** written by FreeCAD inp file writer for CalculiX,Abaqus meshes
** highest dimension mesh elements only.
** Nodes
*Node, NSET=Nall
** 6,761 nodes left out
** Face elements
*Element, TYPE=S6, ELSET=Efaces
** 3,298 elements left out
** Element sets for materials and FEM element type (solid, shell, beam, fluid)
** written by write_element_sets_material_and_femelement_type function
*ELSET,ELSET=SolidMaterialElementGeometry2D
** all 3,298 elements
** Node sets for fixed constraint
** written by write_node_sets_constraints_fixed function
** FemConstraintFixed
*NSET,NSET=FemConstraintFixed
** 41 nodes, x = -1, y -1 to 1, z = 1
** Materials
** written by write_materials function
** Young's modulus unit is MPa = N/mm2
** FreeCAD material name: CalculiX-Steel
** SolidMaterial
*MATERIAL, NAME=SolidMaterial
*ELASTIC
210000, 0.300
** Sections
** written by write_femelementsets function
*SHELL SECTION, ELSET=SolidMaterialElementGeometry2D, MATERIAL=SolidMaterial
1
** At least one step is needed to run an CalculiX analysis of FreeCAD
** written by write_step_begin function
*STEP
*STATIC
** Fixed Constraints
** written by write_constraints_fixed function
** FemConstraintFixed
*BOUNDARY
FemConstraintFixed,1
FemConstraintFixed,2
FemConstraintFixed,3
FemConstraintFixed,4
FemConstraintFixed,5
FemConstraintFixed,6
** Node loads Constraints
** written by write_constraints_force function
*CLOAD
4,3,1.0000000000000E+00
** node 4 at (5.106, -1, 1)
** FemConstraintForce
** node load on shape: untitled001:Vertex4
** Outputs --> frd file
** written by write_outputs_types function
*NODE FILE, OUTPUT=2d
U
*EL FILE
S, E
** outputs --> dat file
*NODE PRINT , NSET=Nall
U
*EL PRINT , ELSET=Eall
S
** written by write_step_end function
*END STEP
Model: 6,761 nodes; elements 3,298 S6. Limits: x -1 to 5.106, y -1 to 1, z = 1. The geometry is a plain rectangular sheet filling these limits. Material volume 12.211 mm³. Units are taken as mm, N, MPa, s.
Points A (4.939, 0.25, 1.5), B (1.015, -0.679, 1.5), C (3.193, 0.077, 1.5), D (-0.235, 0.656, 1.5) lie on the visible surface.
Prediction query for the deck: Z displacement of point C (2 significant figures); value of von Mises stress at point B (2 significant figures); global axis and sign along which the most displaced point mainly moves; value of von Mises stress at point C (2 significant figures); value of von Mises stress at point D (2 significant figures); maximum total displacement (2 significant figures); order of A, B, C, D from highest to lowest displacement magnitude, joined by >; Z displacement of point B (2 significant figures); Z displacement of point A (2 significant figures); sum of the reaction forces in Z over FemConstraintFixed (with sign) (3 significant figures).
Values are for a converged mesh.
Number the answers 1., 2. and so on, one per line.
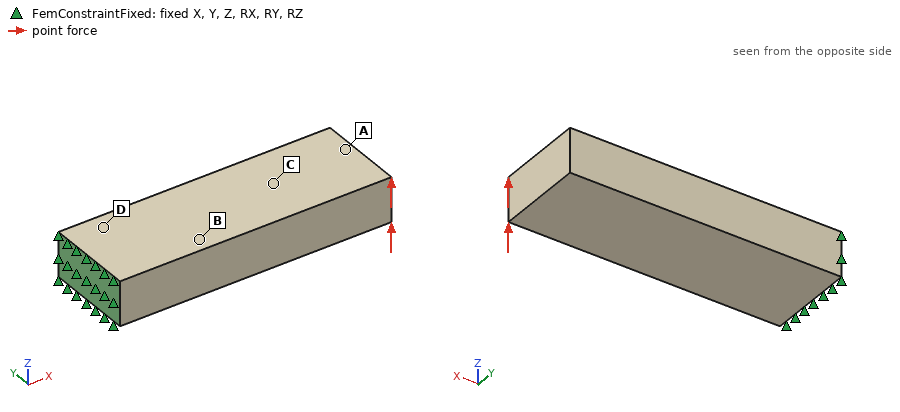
1. 0.0012 mm
2. 13 MPa
3. +Z
4. 6.6 MPa
5. 15 MPa
6. 0.0024 mm
7. A > C > B > D
8. 3.5e-04 mm
9. 0.0020 mm
10. -1.00 N
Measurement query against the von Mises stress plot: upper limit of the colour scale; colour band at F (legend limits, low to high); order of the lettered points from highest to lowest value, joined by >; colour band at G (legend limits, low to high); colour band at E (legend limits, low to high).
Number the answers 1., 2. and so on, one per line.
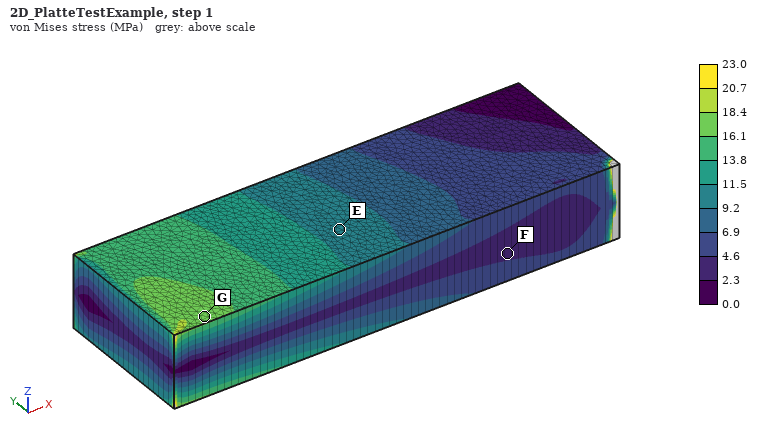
1. 23.0 MPa
2. 2.3 to 4.6 MPa
3. G > E > F
4. 16.1 to 18.4 MPa
5. 9.2 to 11.5 MPa
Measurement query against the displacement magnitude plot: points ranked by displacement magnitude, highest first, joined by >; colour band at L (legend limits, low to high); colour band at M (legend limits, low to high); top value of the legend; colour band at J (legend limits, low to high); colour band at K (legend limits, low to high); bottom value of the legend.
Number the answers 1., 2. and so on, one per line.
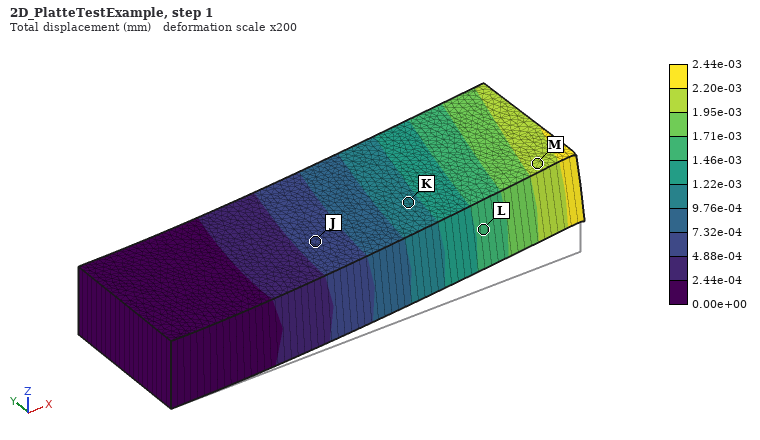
1. M > L > K > J
2. 1.46e-03 to 1.71e-03 mm
3. 1.95e-03 to 2.20e-03 mm
4. 2.44e-03 mm
5. 4.88e-04 to 7.32e-04 mm
6. 9.76e-04 to 1.22e-03 mm
7. 0.00e+00 mm
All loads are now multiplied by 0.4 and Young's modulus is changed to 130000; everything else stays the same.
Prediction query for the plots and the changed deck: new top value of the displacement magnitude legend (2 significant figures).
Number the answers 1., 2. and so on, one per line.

1. 0.0016 mm
